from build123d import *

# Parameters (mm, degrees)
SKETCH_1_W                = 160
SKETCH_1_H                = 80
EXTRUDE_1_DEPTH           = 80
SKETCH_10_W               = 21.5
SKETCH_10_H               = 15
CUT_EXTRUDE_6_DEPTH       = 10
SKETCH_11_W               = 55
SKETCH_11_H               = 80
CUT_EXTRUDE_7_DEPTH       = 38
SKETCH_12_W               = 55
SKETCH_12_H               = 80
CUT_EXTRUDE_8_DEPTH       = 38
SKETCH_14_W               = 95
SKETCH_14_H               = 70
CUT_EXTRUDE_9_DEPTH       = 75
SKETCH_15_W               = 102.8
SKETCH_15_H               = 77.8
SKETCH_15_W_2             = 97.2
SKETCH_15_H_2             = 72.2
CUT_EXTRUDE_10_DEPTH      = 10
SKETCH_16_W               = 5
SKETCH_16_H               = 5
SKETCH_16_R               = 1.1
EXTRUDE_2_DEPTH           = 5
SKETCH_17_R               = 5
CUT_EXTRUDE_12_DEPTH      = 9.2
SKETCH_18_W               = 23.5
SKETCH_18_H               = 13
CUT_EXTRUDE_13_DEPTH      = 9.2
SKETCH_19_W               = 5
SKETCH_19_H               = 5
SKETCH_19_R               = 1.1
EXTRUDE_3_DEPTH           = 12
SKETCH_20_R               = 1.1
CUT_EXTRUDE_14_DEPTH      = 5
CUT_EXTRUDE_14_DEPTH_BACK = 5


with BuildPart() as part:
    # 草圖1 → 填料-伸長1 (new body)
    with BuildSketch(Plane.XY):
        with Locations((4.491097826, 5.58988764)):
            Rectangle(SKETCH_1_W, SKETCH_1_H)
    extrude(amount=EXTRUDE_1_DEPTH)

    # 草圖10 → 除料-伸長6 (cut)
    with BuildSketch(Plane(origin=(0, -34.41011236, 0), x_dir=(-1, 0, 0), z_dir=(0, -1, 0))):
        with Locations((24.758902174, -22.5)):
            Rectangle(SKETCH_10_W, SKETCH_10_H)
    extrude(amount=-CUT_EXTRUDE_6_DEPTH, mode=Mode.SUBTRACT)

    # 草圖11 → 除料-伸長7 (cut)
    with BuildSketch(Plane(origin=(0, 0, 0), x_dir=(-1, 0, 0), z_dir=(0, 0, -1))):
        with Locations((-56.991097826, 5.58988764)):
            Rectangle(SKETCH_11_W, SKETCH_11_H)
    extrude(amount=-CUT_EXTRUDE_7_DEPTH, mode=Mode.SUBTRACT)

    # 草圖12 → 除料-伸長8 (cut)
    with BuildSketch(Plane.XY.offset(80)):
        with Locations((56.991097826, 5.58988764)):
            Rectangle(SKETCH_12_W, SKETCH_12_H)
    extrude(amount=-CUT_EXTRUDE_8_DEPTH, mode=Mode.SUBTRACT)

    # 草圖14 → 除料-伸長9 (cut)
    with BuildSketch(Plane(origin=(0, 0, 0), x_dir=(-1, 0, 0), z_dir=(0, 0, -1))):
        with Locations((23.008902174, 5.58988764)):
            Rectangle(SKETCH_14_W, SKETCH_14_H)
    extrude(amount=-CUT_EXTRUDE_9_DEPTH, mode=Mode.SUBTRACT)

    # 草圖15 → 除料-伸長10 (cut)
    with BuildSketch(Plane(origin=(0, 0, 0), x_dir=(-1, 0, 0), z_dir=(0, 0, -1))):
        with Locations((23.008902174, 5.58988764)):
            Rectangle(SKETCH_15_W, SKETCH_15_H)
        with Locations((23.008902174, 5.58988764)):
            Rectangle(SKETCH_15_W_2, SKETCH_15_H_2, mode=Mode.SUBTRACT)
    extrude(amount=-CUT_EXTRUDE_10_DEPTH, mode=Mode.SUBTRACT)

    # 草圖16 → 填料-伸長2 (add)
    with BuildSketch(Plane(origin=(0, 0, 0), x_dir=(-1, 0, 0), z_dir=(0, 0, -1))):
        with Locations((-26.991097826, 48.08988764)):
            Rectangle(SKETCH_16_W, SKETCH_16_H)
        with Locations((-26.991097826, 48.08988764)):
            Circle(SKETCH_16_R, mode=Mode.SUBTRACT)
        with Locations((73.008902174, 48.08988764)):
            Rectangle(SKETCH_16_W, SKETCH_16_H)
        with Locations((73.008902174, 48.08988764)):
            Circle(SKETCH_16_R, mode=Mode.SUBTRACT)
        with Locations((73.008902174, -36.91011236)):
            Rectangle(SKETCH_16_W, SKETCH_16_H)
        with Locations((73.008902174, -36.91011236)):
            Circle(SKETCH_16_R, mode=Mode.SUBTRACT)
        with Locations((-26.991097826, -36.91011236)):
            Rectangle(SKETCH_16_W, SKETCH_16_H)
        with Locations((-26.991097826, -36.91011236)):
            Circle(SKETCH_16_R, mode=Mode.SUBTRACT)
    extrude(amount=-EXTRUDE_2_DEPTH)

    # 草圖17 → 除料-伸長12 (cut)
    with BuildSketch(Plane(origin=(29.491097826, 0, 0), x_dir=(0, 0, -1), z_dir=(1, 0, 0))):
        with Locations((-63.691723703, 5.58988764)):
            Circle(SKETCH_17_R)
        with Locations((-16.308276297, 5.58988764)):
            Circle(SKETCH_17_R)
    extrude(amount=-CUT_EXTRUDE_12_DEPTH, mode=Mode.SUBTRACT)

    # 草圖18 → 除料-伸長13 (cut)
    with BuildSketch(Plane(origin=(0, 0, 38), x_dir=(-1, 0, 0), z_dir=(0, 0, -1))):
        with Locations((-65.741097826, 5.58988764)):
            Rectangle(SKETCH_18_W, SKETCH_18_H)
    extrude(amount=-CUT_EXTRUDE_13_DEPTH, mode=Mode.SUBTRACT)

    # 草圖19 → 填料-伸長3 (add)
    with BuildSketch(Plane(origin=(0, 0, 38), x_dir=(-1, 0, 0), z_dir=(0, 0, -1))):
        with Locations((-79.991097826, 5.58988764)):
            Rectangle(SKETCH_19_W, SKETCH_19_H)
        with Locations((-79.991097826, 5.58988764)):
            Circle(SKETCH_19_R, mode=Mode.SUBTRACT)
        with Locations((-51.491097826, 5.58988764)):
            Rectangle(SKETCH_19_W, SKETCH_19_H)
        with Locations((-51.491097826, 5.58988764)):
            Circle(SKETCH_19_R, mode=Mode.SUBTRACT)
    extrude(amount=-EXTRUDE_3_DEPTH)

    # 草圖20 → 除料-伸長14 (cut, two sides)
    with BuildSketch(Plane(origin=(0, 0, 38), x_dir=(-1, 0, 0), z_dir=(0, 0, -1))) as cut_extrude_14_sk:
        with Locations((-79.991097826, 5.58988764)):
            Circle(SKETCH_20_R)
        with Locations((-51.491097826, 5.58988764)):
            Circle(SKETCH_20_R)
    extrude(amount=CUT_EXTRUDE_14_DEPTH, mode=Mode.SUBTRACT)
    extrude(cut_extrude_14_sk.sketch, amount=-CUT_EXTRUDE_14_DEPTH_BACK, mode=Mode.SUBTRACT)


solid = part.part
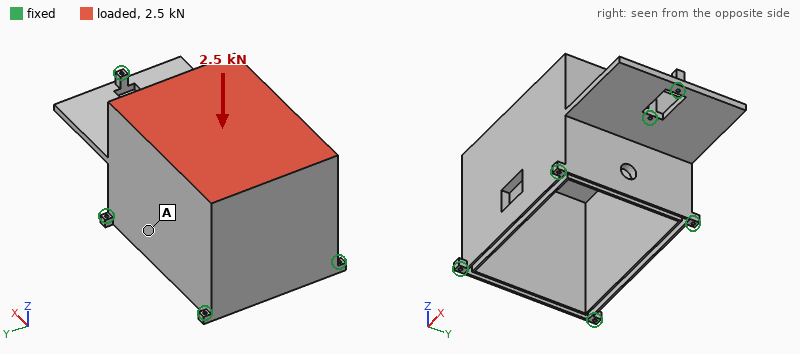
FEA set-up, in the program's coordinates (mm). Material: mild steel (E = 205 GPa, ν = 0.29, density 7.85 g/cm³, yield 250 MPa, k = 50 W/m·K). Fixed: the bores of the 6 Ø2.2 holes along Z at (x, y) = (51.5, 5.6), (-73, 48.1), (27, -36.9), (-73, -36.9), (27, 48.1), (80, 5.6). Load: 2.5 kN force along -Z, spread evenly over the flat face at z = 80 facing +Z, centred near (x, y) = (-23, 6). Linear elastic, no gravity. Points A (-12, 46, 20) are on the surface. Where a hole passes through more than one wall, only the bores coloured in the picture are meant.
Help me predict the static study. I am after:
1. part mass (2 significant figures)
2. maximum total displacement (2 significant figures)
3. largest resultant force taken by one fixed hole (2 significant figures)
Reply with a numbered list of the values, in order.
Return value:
1. 1.4 kg
2. 17 µm
3. 660 N
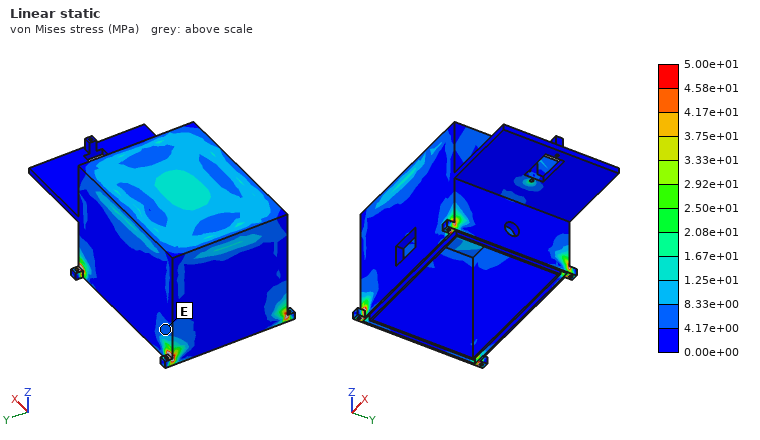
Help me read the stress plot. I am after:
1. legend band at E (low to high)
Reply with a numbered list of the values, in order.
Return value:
1. 4.17e+00 to 8.33e+00 MPa
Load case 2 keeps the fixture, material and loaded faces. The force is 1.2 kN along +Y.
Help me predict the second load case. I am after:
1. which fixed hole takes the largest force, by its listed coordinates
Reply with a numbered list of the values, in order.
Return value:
1. (51.5, 5.6)
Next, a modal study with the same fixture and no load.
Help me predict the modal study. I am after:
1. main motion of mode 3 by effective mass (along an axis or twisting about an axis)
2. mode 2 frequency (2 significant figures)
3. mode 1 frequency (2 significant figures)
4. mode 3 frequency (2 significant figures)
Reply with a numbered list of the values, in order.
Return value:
1. twisting about X
2. 2200 Hz
3. 2200 Hz
4. 2600 Hz
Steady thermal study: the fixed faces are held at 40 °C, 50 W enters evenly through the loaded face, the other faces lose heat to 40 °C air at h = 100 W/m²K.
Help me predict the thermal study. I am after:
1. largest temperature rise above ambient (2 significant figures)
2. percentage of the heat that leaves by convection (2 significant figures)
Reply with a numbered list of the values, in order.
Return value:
1. 23 K
2. 97 %
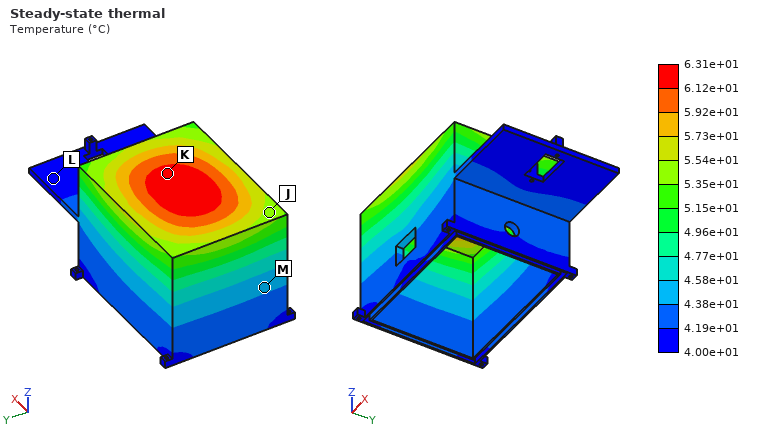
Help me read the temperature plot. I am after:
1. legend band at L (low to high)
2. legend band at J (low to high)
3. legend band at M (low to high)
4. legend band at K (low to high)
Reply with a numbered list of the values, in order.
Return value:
1. 4.00e+01 to 4.19e+01 °C
2. 5.35e+01 to 5.54e+01 °C
3. 4.38e+01 to 4.58e+01 °C
4. 6.12e+01 to 6.31e+01 °C
